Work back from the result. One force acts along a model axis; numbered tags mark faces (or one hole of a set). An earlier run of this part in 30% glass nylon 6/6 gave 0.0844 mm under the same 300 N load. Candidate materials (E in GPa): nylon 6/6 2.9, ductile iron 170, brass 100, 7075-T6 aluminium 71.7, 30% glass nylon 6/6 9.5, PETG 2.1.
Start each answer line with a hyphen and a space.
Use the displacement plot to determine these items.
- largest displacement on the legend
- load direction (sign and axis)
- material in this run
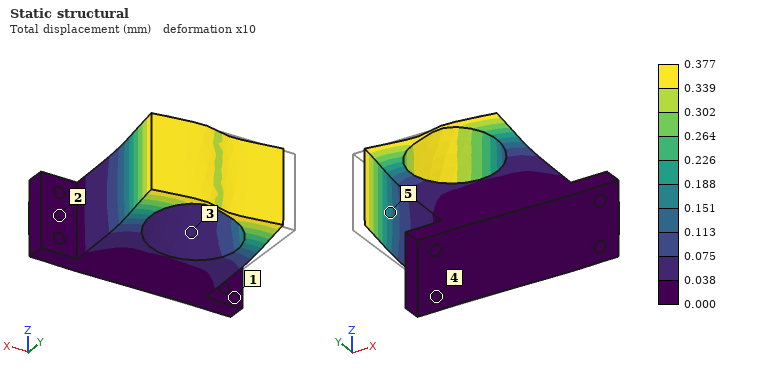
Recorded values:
- 0.377 mm
- +X
- PETG
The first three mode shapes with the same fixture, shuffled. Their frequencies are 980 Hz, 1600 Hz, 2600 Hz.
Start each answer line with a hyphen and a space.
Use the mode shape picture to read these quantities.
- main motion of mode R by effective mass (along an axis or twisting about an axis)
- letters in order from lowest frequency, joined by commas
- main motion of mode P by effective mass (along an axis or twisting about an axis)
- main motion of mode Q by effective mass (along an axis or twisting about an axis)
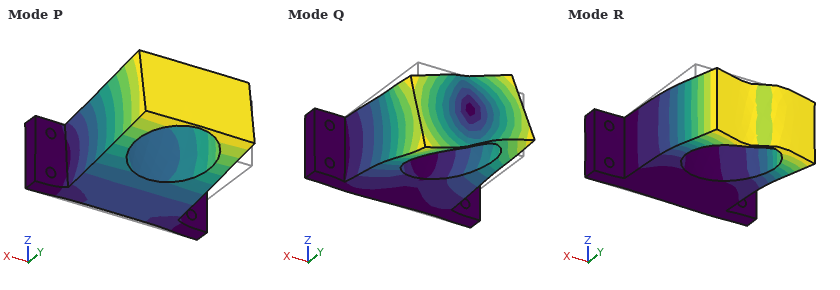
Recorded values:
- along X
- P, R, Q
- along Z
- twisting about Y
